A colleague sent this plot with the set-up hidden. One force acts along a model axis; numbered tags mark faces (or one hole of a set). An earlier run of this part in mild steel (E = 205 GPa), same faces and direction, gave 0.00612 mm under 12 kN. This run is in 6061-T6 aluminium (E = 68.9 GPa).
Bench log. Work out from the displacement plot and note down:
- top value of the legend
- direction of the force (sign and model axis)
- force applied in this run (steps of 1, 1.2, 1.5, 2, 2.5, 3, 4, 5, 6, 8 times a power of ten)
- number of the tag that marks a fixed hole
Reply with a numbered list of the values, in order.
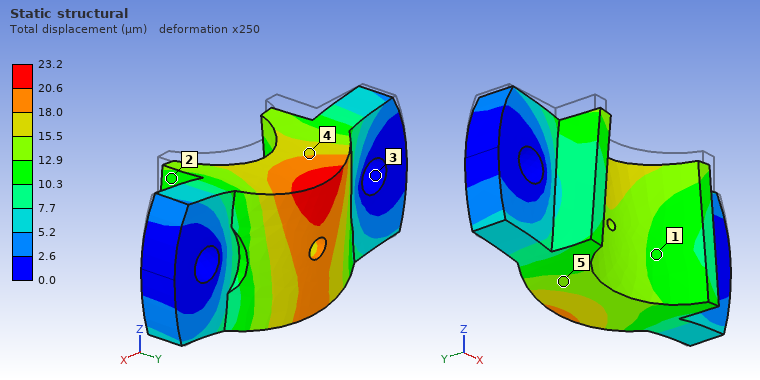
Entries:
1. 23.2 µm
2. -Z
3. 15 kN
4. 3
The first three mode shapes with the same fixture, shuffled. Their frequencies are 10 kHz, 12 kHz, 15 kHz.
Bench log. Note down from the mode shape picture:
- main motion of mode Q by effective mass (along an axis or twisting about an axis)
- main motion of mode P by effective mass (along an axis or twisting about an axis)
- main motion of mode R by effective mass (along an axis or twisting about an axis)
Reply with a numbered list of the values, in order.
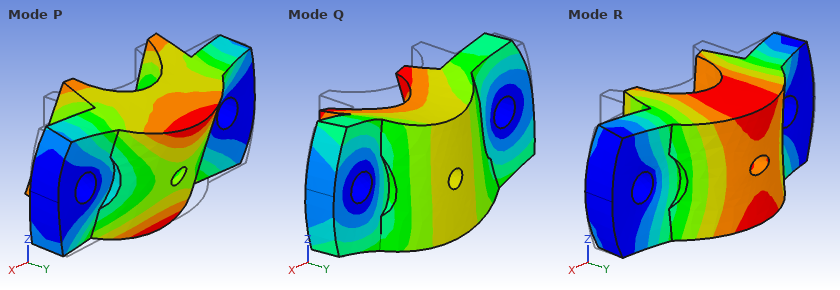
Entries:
1. along Z
2. twisting about X
3. along Y
